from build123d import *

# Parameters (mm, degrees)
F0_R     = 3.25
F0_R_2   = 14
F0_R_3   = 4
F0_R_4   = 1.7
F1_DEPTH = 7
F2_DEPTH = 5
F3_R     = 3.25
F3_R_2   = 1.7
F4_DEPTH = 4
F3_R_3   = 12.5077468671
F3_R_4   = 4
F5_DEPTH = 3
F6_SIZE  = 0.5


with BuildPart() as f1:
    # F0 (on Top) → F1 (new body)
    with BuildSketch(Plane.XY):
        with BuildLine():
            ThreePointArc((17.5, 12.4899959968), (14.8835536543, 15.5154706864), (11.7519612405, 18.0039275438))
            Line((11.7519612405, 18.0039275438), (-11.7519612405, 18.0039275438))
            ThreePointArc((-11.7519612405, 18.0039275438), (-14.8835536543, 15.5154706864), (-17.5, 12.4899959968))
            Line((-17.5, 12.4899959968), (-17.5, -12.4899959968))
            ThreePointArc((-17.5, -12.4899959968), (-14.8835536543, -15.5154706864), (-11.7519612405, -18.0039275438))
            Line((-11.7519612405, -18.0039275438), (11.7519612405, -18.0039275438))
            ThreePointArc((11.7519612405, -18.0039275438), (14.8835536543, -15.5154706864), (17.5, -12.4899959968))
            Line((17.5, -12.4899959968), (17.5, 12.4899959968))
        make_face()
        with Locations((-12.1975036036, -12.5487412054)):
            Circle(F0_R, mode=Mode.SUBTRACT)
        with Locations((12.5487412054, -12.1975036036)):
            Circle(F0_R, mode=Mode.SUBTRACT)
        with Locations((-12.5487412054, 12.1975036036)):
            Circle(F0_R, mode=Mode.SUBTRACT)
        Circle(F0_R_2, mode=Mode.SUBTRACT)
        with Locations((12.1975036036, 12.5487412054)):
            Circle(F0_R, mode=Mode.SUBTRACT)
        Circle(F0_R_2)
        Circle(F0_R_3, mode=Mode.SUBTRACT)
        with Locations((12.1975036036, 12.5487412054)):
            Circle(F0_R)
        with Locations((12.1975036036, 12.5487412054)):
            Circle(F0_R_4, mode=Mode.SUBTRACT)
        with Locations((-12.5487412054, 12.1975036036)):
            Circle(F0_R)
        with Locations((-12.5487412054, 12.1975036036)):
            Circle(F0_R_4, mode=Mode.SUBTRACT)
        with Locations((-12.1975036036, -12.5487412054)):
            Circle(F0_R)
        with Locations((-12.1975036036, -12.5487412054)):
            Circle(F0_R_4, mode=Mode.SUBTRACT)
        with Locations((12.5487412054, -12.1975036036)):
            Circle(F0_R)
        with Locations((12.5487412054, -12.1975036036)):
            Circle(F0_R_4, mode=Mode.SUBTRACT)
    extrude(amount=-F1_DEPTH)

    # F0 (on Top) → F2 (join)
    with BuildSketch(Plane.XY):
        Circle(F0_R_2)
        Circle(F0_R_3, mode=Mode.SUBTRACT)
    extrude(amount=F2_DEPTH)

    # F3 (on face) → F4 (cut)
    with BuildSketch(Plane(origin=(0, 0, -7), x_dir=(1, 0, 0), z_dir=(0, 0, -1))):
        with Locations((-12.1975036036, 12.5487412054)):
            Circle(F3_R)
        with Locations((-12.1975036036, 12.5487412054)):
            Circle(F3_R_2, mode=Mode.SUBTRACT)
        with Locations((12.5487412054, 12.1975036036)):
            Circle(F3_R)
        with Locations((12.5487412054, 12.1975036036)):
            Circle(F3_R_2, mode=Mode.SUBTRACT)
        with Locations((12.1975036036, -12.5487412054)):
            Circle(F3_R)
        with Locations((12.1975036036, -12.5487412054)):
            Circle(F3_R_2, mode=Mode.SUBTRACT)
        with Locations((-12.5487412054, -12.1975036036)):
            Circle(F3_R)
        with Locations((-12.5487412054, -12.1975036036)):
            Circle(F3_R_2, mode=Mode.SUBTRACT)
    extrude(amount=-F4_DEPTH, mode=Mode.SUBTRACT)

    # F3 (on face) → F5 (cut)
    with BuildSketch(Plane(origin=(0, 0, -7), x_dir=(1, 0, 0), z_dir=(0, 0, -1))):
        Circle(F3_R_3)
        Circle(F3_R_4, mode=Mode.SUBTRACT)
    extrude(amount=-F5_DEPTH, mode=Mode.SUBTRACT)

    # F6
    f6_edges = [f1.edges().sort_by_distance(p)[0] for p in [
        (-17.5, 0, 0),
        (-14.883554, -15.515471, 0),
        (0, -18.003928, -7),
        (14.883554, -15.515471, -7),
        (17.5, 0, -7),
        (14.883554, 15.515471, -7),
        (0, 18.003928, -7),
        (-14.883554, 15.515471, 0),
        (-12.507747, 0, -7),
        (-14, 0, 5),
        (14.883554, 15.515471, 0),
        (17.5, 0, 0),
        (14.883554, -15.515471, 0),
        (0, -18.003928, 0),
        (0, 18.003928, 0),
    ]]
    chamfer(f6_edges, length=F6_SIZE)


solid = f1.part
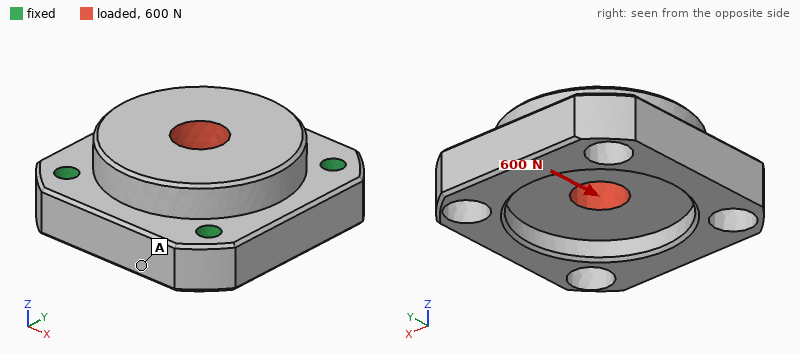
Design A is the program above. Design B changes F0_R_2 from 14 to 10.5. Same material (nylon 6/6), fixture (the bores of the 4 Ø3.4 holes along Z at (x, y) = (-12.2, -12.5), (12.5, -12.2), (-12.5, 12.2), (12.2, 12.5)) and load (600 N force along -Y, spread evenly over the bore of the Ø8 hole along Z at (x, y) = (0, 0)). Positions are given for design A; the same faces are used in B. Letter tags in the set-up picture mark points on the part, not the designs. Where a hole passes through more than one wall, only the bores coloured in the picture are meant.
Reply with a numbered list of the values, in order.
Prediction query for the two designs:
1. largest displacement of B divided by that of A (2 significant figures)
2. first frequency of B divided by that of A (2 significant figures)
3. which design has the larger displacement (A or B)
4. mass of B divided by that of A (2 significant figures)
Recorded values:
1. 1.4
2. 0.94
3. B
4. 0.85
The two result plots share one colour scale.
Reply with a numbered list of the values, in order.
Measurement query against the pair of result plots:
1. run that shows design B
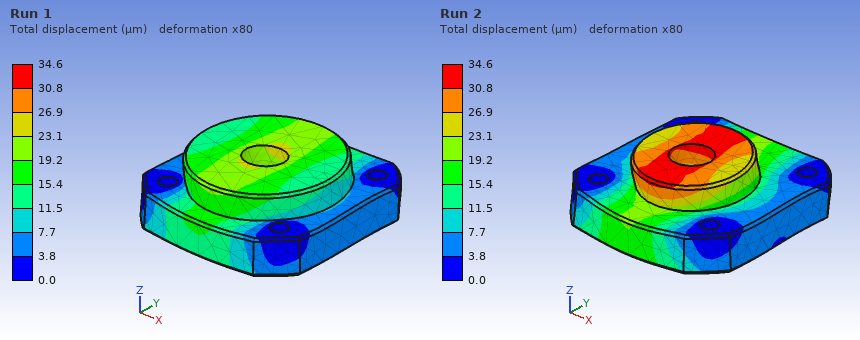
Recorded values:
1. Run 2
